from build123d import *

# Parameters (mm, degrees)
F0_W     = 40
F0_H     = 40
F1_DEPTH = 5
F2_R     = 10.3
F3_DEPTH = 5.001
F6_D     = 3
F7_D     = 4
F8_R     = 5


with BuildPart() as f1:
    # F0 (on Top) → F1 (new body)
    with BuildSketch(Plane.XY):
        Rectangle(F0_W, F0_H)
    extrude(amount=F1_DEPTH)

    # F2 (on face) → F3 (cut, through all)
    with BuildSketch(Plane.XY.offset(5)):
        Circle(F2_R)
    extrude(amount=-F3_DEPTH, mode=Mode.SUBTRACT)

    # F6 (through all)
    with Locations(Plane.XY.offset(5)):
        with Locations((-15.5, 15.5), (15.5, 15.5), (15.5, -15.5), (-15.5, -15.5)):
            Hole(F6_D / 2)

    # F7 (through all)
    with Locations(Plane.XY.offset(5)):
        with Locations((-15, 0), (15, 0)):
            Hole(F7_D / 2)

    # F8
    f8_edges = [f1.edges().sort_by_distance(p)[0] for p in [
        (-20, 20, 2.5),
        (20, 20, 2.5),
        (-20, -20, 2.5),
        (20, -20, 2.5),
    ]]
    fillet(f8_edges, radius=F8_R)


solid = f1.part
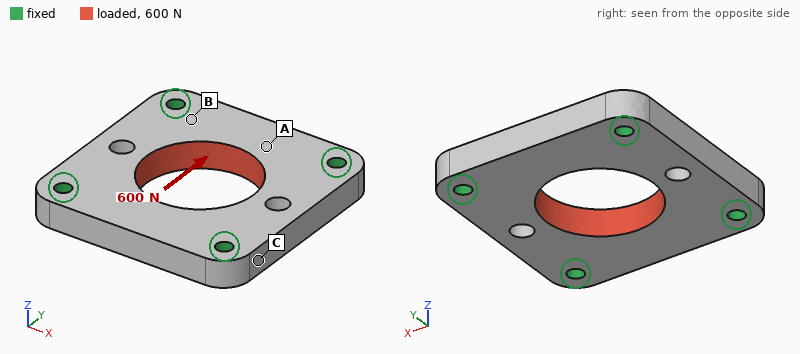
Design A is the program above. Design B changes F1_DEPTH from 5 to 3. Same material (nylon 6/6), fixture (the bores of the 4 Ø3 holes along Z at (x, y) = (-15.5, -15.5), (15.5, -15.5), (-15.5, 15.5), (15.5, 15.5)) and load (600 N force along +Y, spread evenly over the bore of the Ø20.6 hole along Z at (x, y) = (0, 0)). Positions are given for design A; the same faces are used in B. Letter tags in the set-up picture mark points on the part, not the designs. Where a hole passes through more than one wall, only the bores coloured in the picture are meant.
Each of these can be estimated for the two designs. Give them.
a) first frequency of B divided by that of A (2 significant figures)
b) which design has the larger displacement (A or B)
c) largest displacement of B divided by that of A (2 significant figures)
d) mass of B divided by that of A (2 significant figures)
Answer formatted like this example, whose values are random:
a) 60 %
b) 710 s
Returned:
a) 0.70
b) B
c) 1.7
d) 0.60
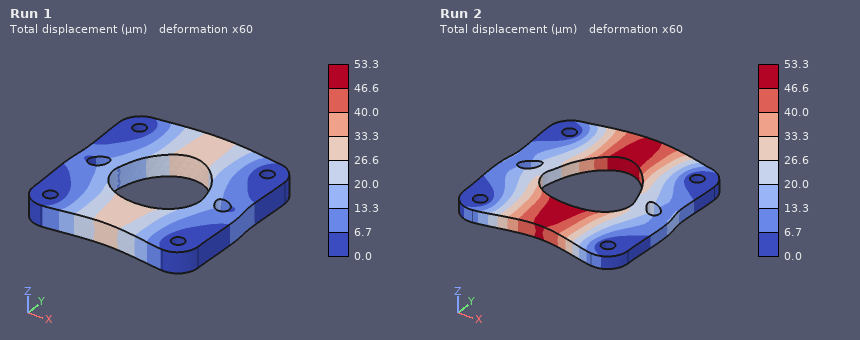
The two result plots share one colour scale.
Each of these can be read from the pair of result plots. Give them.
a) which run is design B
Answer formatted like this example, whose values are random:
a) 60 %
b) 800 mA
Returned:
a) Run 2
